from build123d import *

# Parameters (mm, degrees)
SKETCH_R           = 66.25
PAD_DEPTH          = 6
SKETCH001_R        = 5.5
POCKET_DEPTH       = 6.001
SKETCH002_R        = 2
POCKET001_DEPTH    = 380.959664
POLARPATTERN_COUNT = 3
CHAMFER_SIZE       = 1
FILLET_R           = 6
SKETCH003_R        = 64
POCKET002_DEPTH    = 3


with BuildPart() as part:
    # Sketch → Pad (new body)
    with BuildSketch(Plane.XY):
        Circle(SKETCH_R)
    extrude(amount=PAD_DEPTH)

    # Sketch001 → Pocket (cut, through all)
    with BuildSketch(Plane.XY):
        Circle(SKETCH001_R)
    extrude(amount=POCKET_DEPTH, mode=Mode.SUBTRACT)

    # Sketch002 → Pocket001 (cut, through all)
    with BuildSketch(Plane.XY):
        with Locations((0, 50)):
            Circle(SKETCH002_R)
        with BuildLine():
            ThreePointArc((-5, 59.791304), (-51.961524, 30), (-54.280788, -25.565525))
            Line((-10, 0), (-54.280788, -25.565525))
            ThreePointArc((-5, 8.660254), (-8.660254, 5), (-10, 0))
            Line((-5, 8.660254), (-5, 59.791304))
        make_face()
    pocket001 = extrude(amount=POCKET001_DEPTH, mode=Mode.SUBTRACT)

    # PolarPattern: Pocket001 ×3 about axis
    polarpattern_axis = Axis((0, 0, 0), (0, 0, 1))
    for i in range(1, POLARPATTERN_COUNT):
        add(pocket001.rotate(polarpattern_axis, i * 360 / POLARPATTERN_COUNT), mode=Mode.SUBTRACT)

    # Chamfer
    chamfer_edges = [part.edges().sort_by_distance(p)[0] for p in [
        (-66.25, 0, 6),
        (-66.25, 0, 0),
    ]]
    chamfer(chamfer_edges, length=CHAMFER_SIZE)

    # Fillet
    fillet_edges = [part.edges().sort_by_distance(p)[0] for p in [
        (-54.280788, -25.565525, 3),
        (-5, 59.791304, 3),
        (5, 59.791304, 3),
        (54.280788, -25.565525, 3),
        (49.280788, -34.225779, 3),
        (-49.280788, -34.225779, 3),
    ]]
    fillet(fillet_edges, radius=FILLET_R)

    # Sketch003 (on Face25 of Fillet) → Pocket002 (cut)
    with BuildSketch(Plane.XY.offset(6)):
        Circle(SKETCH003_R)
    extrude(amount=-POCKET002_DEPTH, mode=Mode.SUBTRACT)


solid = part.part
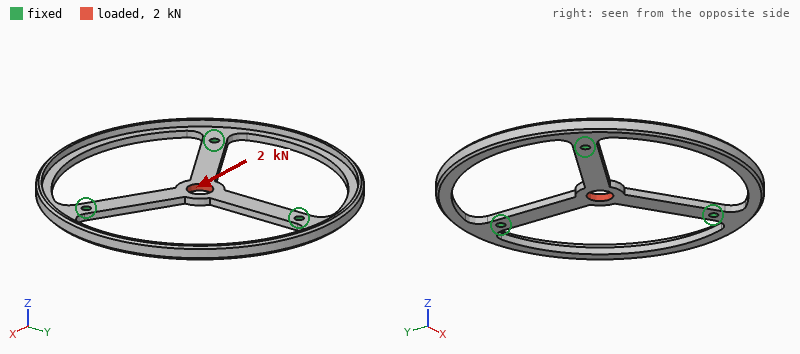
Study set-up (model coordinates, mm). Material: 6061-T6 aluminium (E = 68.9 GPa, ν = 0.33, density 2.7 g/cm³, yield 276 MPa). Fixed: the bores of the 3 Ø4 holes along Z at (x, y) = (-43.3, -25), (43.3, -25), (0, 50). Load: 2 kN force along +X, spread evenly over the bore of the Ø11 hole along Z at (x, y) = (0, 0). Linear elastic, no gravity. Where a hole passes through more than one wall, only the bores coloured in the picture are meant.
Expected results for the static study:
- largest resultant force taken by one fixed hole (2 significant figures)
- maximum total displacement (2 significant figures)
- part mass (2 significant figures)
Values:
1.2 kN
53 µm
41 g
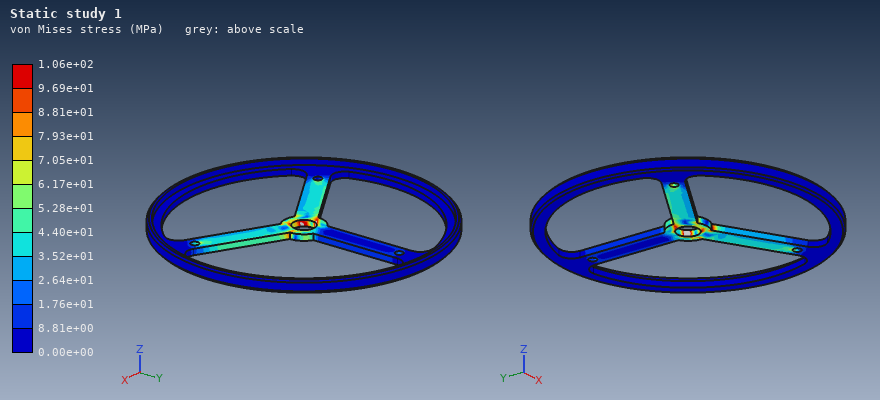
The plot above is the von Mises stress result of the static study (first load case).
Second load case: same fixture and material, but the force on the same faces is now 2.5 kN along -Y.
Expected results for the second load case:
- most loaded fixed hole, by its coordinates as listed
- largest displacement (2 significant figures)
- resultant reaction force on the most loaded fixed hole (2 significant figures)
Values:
(0, 50)
69 µm
1.7 kN
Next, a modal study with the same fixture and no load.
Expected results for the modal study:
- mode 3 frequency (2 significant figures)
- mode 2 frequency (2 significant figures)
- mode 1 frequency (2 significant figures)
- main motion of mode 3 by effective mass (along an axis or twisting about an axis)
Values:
1400 Hz
910 Hz
910 Hz
along Z
